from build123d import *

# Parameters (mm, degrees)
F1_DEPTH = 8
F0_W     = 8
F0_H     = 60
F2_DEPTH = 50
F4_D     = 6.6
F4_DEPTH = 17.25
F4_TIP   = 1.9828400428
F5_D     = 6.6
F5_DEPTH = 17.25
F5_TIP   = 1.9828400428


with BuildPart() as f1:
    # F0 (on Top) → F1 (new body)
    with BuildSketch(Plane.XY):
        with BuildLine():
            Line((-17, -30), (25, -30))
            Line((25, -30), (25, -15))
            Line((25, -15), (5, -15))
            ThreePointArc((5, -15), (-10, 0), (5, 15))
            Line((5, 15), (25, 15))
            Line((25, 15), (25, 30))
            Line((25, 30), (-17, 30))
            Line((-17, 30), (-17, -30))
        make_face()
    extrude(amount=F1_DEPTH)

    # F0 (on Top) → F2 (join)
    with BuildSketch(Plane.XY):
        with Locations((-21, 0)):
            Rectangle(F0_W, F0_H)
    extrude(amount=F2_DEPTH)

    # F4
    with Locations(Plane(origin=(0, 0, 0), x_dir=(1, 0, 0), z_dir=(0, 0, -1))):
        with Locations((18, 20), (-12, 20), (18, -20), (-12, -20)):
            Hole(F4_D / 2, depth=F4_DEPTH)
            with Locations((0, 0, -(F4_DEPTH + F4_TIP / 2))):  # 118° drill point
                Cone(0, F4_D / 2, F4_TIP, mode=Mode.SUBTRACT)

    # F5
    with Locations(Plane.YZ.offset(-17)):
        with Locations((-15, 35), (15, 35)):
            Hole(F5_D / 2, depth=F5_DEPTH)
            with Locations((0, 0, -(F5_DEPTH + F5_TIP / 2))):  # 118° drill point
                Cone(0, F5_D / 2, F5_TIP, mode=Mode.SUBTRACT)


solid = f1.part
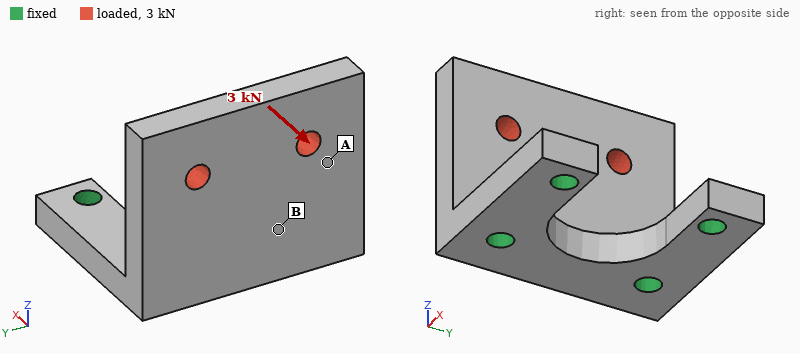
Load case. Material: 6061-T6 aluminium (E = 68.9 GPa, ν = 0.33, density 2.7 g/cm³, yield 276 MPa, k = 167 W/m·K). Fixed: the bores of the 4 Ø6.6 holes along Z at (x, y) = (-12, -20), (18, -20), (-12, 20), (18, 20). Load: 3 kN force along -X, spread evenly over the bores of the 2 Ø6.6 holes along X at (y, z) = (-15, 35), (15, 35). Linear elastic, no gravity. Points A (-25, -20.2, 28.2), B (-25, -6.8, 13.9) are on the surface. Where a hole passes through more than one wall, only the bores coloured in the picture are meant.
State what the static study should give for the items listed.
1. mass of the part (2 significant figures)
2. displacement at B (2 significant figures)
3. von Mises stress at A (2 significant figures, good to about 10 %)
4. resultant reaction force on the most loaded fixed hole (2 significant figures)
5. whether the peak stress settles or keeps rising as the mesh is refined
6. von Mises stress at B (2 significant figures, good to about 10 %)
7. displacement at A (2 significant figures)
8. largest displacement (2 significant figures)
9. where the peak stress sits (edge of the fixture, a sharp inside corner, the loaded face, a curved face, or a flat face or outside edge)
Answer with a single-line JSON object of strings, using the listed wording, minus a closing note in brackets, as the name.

{"mass of the part": "94 g", "displacement at B": "0.089 mm", "von Mises stress at A": "37 MPa", "resultant reaction force on the most loaded fixed hole": "1.6 kN", "whether the peak stress settles or keeps rising as the mesh is refined": "keeps rising", "von Mises stress at B": "84 MPa", "displacement at A": "0.22 mm", "largest displacement": "0.47 mm", "where the peak stress sits": "edge of the fixture"}
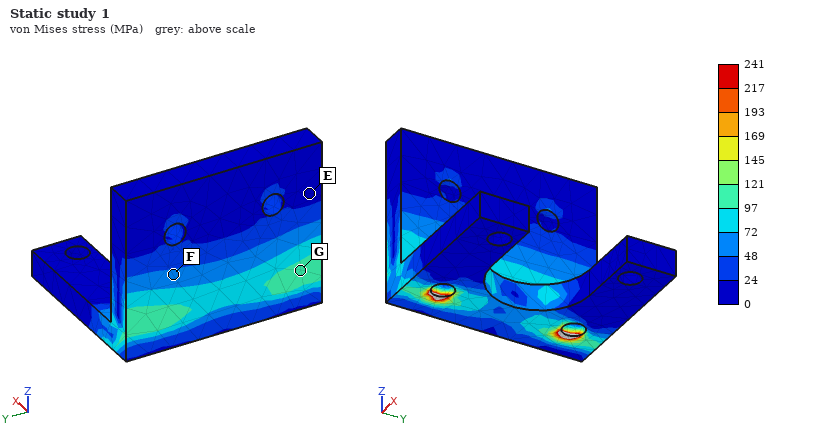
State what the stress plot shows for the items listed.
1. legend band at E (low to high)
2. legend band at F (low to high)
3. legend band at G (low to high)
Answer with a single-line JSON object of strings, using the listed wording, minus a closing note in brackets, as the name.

{"legend band at E": "0 to 24 MPa", "legend band at F": "48 to 72 MPa", "legend band at G": "97 to 121 MPa"}
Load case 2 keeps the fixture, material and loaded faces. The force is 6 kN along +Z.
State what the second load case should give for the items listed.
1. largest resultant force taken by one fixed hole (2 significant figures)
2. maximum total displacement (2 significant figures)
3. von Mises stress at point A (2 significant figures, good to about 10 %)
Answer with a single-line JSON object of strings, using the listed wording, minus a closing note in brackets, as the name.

{"largest resultant force taken by one fixed hole": "3.1 kN", "maximum total displacement": "84 µm", "von Mises stress at point A": "17 MPa"}
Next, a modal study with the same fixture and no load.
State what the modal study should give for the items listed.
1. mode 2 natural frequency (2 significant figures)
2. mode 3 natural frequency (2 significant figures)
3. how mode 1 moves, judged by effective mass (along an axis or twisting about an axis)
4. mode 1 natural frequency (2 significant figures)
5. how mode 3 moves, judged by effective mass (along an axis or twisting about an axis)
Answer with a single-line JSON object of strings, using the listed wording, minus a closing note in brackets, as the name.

{"mode 2 natural frequency": "5300 Hz", "mode 3 natural frequency": "8600 Hz", "how mode 1 moves, judged by effective mass": "along X", "mode 1 natural frequency": "2400 Hz", "how mode 3 moves, judged by effective mass": "along Y"}
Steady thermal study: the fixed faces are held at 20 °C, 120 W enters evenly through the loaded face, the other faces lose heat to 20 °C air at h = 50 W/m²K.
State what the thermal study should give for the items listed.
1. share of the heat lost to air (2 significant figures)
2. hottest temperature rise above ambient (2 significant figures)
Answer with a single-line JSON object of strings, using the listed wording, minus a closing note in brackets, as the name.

{"share of the heat lost to air": "11 %", "hottest temperature rise above ambient": "60 K"}
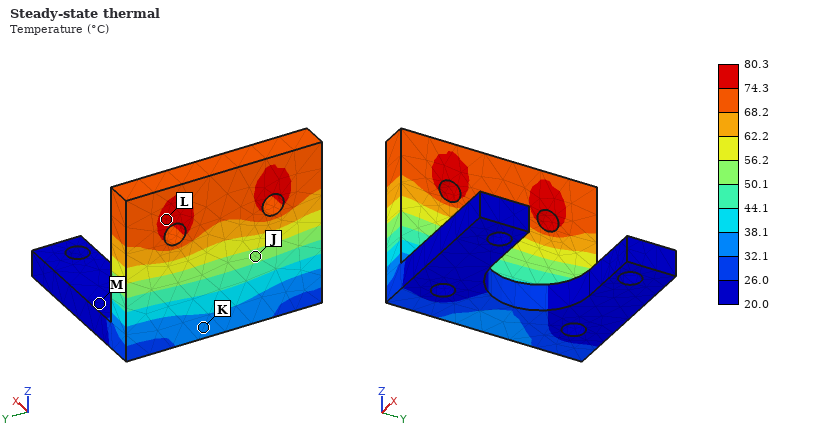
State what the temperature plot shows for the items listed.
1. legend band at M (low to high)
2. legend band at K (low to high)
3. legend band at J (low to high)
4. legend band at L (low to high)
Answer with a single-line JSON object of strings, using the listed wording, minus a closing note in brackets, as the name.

{"legend band at M": "20.0 to 26.0 °C", "legend band at K": "32.1 to 38.1 °C", "legend band at J": "50.1 to 56.2 °C", "legend band at L": "74.3 to 80.3 °C"}
